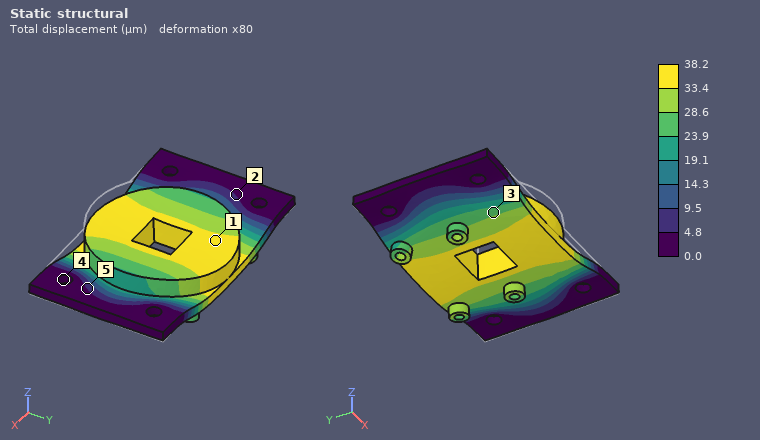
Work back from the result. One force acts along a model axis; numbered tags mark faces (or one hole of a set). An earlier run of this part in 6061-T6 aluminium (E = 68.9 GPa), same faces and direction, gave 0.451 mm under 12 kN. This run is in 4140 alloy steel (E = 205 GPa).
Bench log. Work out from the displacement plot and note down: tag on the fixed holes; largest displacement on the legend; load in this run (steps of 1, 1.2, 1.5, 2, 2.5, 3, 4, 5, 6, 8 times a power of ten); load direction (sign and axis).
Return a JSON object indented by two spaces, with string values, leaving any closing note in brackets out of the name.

{
  "tag on the fixed holes": "4",
  "largest displacement on the legend": "38.2 µm",
  "load in this run": "3 kN",
  "load direction": "-Z"
}
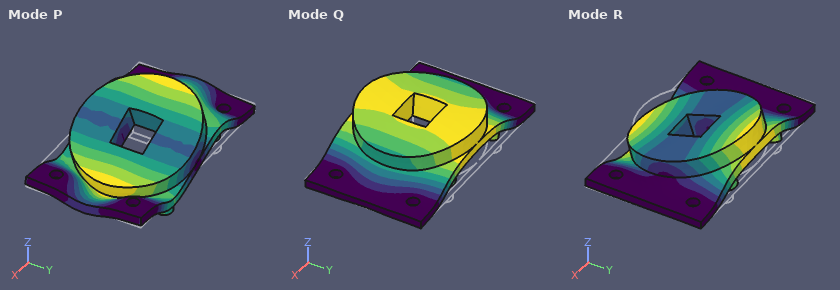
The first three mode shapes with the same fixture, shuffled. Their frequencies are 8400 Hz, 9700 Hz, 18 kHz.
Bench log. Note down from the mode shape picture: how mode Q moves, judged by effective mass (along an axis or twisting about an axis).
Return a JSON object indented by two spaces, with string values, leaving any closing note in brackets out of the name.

{
  "how mode Q moves, judged by effective mass": "along Z"
}
